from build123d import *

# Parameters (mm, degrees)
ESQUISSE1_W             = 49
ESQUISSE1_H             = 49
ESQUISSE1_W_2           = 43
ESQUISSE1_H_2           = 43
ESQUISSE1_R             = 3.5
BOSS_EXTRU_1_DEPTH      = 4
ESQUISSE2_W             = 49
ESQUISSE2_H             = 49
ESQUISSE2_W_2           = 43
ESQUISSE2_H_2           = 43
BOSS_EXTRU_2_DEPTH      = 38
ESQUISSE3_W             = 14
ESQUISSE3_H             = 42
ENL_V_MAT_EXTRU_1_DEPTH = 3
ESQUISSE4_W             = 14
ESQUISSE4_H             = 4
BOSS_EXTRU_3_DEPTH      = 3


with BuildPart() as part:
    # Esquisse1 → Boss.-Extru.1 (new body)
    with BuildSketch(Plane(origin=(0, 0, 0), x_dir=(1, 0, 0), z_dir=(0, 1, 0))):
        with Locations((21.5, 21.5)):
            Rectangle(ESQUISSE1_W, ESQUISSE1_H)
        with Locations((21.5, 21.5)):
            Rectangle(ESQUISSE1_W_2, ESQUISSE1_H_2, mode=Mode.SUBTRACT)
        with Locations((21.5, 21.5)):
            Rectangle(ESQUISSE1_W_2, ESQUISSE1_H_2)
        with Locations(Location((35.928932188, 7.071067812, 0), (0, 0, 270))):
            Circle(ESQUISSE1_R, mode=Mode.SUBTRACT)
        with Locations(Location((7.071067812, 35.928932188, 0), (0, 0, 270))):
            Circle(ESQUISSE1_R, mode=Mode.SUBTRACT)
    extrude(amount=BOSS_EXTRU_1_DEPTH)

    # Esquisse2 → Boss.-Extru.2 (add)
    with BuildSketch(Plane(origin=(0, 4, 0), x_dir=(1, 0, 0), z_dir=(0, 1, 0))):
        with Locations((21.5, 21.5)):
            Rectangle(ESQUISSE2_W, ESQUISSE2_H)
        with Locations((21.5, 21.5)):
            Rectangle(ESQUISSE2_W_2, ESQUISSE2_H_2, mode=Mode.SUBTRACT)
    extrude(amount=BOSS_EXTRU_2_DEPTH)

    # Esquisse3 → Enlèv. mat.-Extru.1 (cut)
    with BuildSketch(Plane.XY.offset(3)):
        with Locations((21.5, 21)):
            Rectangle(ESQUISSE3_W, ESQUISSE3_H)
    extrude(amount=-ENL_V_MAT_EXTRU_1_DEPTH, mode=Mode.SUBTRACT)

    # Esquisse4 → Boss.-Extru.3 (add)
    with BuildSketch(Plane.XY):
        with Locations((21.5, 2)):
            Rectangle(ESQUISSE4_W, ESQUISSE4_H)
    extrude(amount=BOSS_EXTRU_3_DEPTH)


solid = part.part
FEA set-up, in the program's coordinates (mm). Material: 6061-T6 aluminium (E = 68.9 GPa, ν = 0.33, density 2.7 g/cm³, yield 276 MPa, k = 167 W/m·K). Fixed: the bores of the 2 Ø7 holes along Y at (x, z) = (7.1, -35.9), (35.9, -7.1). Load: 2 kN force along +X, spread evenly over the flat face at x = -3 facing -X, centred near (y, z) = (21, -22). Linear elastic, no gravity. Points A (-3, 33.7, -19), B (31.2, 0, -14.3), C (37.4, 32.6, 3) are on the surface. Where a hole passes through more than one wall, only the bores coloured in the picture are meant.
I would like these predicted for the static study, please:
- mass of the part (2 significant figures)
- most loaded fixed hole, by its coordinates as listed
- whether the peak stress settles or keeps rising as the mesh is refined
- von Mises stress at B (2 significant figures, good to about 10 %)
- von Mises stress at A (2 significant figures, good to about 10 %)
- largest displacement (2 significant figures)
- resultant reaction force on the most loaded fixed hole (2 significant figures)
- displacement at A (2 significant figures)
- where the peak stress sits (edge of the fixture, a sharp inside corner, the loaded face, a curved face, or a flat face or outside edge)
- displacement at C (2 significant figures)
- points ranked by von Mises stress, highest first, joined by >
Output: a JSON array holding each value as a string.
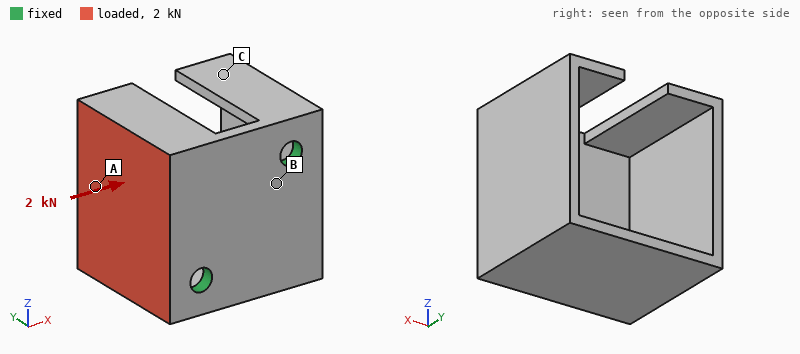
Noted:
["77 g", "(7.1, -35.9)", "keeps rising", "42 MPa", "78 MPa", "0.55 mm", "1.3 kN", "0.40 mm", "edge of the fixture", "0.12 mm", "A > B > C"]
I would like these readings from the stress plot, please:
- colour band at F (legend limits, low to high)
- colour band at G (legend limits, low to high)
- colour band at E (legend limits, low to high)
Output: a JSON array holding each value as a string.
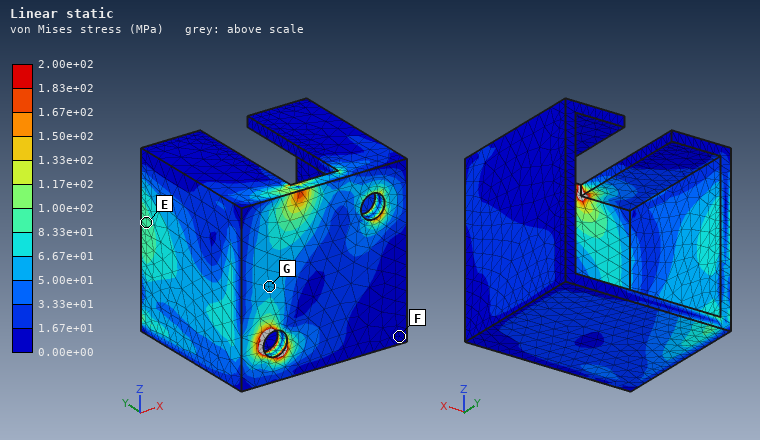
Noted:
["0.00e+00 to 1.67e+01 MPa", "5.00e+01 to 6.67e+01 MPa", "8.33e+01 to 1.00e+02 MPa"]
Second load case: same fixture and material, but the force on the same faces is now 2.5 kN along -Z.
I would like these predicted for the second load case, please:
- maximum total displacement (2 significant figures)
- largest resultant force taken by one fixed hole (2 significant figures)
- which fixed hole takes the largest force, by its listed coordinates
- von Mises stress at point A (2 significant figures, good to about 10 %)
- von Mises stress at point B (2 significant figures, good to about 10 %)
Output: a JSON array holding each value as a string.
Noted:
["0.54 mm", "2.6 kN", "(7.1, -35.9)", "31 MPa", "41 MPa"]
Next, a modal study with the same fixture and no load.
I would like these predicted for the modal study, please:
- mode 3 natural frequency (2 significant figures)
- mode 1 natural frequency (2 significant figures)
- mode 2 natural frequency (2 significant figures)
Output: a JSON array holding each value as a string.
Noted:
["3300 Hz", "1900 Hz", "2300 Hz"]
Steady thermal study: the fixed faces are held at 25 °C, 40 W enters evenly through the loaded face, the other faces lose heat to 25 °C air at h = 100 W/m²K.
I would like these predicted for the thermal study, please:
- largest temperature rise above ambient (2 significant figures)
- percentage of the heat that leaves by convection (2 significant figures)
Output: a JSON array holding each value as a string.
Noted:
["26 K", "30 %"]
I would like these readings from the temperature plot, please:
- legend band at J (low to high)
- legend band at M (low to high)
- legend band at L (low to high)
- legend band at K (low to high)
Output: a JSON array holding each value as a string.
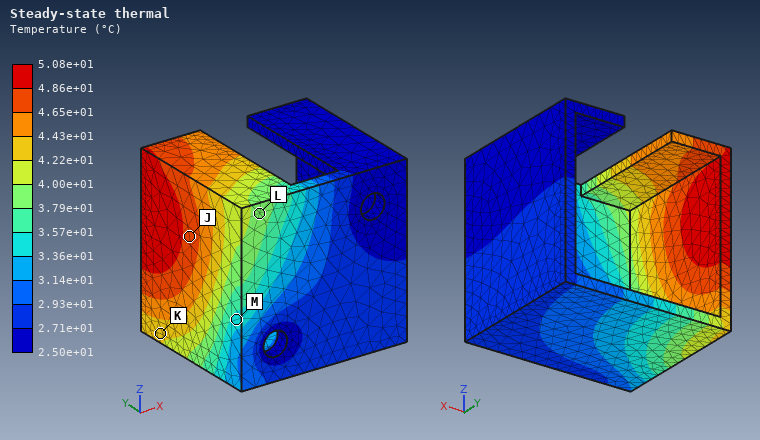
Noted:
["4.65e+01 to 4.86e+01 °C", "3.36e+01 to 3.57e+01 °C", "3.79e+01 to 4.00e+01 °C", "4.22e+01 to 4.43e+01 °C"]
